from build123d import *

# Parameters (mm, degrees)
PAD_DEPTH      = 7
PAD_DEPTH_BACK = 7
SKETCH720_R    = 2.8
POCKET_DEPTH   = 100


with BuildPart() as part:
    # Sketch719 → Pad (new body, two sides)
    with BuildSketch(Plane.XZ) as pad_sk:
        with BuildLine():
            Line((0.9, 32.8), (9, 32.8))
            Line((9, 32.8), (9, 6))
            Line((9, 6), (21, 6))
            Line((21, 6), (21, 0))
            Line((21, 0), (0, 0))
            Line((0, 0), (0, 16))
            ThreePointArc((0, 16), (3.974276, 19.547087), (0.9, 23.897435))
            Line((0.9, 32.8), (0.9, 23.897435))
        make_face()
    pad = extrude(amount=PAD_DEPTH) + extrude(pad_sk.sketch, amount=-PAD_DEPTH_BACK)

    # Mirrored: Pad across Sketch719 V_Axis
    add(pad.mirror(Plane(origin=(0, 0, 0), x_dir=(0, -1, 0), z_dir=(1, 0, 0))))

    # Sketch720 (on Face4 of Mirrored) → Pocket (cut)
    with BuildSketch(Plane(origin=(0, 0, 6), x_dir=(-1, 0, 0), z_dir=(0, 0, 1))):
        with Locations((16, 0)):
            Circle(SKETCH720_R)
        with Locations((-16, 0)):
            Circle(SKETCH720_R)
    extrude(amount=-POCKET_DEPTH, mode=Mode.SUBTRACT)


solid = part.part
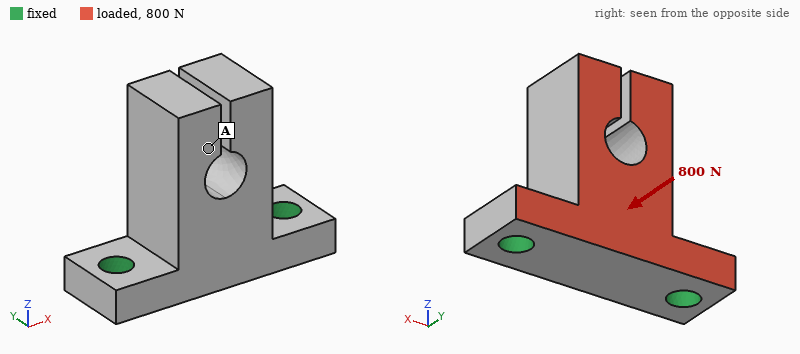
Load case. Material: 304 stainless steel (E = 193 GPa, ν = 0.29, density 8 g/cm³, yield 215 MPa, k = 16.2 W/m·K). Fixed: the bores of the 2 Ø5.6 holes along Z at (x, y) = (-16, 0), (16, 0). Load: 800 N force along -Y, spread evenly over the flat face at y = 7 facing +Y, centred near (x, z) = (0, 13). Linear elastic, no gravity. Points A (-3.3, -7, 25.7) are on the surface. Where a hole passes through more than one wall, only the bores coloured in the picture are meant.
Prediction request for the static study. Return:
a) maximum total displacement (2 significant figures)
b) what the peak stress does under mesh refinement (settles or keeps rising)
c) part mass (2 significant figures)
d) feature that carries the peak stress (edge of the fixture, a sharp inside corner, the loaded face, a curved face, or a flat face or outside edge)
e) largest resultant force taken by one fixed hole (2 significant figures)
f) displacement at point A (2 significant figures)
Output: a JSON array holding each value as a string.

["17 µm", "keeps rising", "72 g", "edge of the fixture", "400 N", "13 µm"]
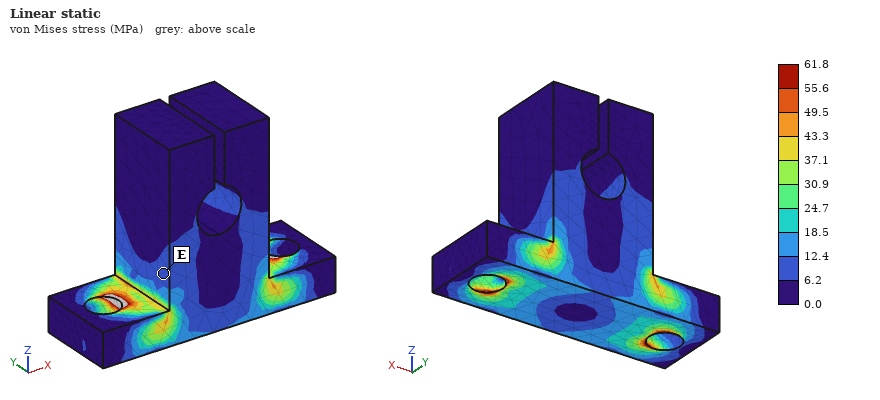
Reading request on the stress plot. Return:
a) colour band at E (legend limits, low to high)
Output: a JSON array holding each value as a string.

["6.2 to 12.4 MPa"]
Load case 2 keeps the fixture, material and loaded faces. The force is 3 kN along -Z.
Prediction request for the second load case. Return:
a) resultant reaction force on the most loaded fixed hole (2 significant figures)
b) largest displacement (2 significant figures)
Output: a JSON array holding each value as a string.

["1.6 kN", "36 µm"]
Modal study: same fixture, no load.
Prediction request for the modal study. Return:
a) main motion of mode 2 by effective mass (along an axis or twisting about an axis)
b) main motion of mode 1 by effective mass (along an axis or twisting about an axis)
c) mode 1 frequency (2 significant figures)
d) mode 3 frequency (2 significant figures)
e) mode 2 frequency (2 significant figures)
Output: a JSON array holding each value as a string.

["along X", "along Y", "4900 Hz", "9500 Hz", "7800 Hz"]
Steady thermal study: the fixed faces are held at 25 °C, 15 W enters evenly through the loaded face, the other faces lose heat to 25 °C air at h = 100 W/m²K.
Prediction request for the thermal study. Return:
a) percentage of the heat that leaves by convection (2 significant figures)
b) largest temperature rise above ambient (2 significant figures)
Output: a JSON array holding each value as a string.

["43 %", "37 K"]
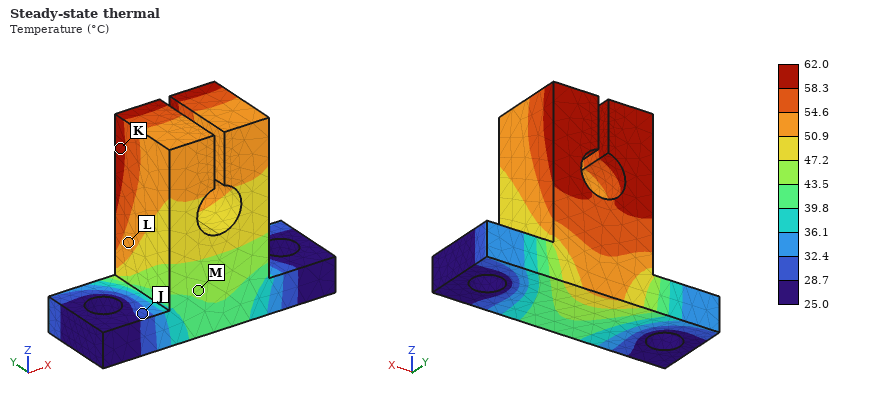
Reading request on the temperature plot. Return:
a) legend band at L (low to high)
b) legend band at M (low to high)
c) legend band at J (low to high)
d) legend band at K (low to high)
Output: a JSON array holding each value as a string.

["50.9 to 54.6 °C", "43.5 to 47.2 °C", "28.7 to 32.4 °C", "58.3 to 62.0 °C"]
